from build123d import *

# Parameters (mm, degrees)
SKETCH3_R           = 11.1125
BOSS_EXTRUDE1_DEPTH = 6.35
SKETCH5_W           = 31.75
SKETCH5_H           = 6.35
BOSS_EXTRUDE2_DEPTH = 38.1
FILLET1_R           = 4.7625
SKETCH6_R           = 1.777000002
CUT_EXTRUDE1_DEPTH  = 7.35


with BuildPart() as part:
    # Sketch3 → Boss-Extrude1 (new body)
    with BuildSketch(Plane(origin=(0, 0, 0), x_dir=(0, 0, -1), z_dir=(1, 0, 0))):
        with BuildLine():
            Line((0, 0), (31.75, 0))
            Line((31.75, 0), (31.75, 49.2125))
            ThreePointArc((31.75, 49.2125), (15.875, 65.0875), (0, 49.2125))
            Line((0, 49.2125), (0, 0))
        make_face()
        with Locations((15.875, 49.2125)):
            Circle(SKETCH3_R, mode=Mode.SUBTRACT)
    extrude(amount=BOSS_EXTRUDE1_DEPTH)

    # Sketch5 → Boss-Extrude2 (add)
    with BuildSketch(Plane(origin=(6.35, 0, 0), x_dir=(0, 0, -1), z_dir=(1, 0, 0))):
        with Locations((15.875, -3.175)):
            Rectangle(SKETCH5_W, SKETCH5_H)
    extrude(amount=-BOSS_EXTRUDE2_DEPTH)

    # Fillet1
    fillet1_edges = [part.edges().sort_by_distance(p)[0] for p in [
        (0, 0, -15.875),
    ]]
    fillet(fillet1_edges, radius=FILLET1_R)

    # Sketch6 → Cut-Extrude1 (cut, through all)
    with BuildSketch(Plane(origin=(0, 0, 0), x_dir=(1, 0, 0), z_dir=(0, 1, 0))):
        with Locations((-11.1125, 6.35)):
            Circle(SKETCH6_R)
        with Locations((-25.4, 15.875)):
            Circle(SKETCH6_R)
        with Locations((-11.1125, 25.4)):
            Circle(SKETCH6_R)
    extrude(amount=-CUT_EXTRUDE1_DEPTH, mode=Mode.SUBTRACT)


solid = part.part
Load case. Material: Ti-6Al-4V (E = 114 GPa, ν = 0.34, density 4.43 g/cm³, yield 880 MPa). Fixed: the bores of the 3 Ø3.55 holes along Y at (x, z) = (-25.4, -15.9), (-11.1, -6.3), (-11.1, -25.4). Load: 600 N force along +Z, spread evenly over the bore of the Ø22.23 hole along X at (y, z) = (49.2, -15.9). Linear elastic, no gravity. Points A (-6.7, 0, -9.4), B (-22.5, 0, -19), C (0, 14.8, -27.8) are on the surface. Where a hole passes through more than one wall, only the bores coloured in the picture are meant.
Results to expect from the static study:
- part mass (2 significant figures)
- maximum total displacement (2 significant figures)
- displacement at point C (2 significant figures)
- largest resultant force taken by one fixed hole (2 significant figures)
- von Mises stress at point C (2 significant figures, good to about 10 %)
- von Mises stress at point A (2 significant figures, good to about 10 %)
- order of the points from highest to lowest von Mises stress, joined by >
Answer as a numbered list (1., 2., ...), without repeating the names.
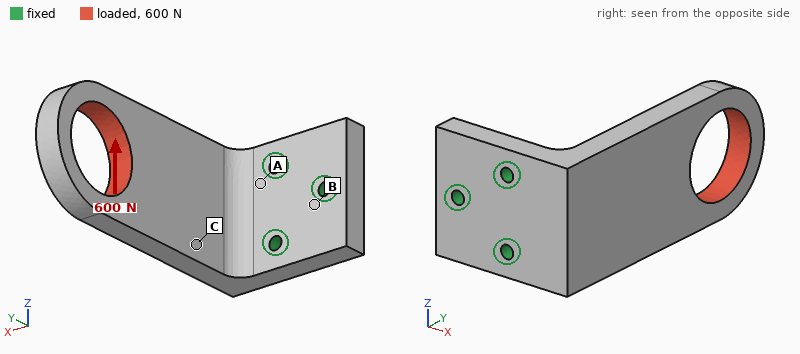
1. 78 g
2. 0.13 mm
3. 0.036 mm
4. 1.5 kN
5. 24 MPa
6. 54 MPa
7. A > C > B
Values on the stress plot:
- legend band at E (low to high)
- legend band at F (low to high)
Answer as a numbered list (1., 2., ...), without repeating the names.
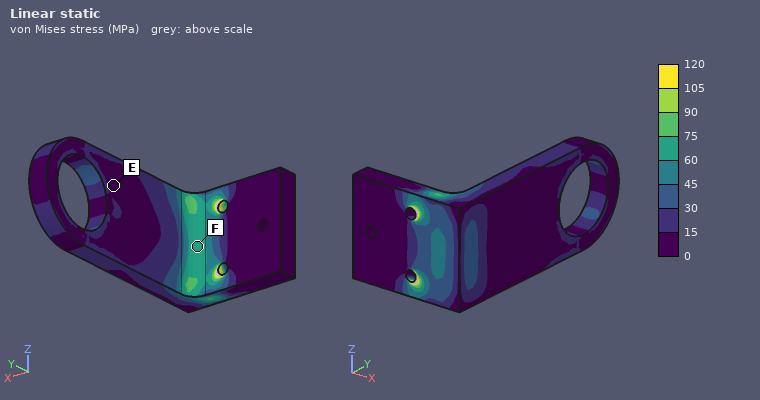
1. 0 to 15 MPa
2. 60 to 75 MPa
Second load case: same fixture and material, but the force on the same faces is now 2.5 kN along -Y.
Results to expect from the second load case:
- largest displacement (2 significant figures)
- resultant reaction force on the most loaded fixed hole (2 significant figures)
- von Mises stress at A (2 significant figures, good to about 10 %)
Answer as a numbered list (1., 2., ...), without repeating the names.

1. 0.23 mm
2. 1.5 kN
3. 110 MPa
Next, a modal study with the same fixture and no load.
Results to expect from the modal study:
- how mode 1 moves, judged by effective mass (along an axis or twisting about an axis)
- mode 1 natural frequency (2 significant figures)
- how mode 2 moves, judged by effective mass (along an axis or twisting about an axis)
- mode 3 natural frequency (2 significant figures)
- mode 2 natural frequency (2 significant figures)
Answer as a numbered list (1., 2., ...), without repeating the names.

1. along X
2. 1300 Hz
3. along Z
4. 5200 Hz
5. 2800 Hz
